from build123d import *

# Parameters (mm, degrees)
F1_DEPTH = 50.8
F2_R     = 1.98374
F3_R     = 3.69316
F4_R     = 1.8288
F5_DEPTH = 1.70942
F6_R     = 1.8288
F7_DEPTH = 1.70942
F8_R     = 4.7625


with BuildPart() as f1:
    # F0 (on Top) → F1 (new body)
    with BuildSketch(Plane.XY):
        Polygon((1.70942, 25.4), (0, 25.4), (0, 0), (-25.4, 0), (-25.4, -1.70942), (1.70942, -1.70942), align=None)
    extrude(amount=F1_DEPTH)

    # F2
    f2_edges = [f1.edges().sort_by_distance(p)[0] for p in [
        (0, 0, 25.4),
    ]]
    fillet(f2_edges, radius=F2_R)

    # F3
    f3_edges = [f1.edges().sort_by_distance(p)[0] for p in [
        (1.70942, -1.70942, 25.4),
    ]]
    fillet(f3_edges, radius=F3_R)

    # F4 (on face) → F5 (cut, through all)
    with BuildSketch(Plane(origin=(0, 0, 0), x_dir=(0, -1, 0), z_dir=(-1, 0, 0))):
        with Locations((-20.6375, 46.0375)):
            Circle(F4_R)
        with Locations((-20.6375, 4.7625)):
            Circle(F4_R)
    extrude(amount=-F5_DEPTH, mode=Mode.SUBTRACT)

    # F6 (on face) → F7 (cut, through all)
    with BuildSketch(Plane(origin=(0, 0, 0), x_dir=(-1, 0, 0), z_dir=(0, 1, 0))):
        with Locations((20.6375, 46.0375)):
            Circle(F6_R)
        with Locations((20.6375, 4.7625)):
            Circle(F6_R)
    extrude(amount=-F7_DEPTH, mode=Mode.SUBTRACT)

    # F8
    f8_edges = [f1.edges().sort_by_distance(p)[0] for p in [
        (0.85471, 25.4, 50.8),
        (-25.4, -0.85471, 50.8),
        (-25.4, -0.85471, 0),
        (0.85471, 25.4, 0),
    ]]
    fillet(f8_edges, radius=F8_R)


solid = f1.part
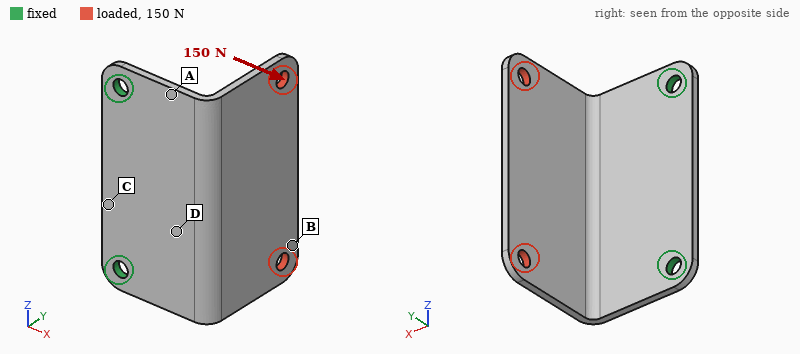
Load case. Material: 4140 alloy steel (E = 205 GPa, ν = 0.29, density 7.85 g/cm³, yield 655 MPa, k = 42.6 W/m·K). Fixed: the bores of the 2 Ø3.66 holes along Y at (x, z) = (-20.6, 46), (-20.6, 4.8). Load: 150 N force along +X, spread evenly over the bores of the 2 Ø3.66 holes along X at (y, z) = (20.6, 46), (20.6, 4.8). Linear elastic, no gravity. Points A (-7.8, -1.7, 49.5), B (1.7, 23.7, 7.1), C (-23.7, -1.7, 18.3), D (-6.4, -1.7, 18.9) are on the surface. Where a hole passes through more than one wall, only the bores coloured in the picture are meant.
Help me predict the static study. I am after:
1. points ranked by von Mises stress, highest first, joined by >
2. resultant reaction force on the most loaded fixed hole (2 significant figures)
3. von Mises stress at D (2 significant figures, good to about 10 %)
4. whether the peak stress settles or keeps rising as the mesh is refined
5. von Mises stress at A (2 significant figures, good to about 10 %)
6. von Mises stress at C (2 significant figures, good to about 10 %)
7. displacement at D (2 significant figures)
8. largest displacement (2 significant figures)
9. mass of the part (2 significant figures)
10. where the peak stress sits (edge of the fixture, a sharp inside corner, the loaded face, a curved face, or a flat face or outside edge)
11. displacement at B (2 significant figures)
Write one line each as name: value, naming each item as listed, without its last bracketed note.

points ranked by von Mises stress, highest first, joined by >: A > D > C > B
resultant reaction force on the most loaded fixed hole: 80 N
von Mises stress at D: 110 MPa
whether the peak stress settles or keeps rising as the mesh is refined: keeps rising
von Mises stress at A: 150 MPa
von Mises stress at C: 59 MPa
displacement at D: 0.100 mm
largest displacement: 0.63 mm
mass of the part: 34 g
where the peak stress sits: edge of the fixture
displacement at B: 0.58 mm
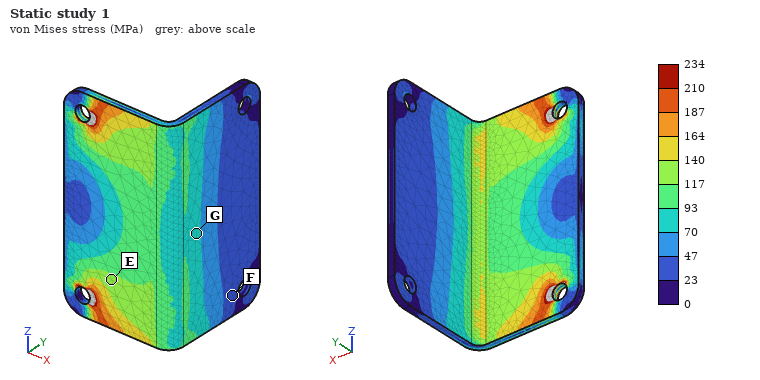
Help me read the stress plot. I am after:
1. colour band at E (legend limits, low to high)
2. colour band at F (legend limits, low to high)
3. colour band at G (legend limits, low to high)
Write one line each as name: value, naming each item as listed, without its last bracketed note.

colour band at E: 117 to 140 MPa
colour band at F: 23 to 47 MPa
colour band at G: 70 to 93 MPa
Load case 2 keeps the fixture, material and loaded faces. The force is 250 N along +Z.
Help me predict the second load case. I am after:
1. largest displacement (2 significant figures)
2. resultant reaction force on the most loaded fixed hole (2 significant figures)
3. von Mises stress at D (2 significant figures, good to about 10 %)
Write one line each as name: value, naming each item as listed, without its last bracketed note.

largest displacement: 0.21 mm
resultant reaction force on the most loaded fixed hole: 220 N
von Mises stress at D: 72 MPa
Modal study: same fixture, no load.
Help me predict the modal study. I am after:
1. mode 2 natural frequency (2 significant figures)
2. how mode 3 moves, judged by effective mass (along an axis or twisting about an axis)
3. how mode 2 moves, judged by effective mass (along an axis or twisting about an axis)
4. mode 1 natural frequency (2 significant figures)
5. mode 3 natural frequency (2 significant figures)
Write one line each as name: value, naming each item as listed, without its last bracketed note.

mode 2 natural frequency: 1600 Hz
how mode 3 moves, judged by effective mass: along Y
how mode 2 moves, judged by effective mass: along Z
mode 1 natural frequency: 800 Hz
mode 3 natural frequency: 2200 Hz
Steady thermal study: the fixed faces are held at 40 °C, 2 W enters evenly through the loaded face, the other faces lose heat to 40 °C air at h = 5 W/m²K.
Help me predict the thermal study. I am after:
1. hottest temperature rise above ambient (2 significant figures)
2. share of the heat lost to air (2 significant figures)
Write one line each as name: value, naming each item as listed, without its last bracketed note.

hottest temperature rise above ambient: 29 K
share of the heat lost to air: 17 %
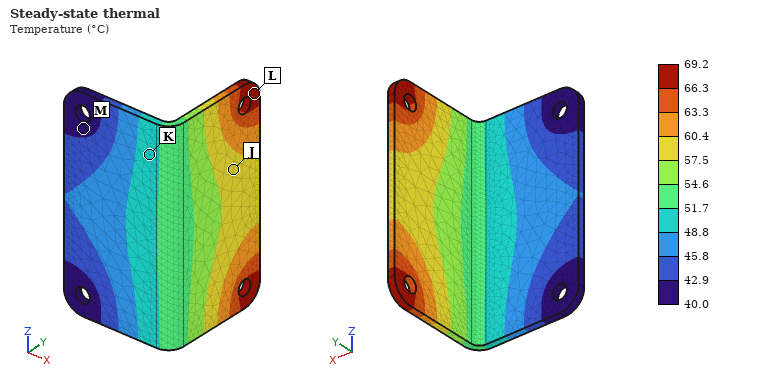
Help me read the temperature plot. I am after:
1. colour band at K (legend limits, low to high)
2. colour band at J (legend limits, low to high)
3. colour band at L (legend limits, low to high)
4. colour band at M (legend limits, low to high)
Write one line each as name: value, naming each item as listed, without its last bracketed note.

colour band at K: 48.8 to 51.7 °C
colour band at J: 57.5 to 60.4 °C
colour band at L: 66.3 to 69.2 °C
colour band at M: 40.0 to 42.9 °C
